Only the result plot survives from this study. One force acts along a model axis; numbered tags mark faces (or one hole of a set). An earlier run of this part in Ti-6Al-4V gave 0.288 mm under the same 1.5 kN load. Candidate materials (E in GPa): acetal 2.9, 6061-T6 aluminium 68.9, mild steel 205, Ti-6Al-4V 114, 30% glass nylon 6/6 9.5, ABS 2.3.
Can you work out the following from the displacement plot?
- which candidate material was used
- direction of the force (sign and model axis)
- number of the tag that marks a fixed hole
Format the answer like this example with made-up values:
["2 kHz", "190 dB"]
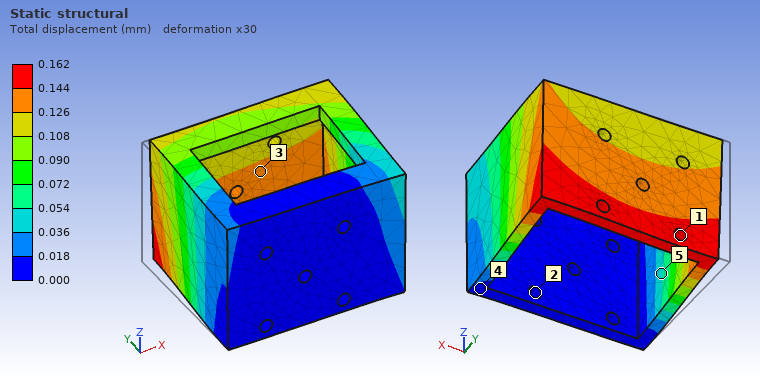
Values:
["mild steel", "+X", "2"]
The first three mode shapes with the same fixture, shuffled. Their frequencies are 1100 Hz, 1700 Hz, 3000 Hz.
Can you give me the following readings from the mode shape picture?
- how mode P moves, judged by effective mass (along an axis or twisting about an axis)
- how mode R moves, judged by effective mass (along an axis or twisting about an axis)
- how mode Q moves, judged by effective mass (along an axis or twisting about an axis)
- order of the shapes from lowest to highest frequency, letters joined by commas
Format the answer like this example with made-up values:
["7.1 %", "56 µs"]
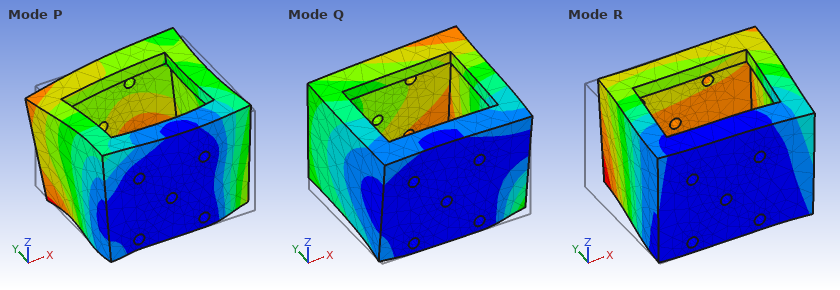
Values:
["along Y", "along X", "along Z", "R, Q, P"]
